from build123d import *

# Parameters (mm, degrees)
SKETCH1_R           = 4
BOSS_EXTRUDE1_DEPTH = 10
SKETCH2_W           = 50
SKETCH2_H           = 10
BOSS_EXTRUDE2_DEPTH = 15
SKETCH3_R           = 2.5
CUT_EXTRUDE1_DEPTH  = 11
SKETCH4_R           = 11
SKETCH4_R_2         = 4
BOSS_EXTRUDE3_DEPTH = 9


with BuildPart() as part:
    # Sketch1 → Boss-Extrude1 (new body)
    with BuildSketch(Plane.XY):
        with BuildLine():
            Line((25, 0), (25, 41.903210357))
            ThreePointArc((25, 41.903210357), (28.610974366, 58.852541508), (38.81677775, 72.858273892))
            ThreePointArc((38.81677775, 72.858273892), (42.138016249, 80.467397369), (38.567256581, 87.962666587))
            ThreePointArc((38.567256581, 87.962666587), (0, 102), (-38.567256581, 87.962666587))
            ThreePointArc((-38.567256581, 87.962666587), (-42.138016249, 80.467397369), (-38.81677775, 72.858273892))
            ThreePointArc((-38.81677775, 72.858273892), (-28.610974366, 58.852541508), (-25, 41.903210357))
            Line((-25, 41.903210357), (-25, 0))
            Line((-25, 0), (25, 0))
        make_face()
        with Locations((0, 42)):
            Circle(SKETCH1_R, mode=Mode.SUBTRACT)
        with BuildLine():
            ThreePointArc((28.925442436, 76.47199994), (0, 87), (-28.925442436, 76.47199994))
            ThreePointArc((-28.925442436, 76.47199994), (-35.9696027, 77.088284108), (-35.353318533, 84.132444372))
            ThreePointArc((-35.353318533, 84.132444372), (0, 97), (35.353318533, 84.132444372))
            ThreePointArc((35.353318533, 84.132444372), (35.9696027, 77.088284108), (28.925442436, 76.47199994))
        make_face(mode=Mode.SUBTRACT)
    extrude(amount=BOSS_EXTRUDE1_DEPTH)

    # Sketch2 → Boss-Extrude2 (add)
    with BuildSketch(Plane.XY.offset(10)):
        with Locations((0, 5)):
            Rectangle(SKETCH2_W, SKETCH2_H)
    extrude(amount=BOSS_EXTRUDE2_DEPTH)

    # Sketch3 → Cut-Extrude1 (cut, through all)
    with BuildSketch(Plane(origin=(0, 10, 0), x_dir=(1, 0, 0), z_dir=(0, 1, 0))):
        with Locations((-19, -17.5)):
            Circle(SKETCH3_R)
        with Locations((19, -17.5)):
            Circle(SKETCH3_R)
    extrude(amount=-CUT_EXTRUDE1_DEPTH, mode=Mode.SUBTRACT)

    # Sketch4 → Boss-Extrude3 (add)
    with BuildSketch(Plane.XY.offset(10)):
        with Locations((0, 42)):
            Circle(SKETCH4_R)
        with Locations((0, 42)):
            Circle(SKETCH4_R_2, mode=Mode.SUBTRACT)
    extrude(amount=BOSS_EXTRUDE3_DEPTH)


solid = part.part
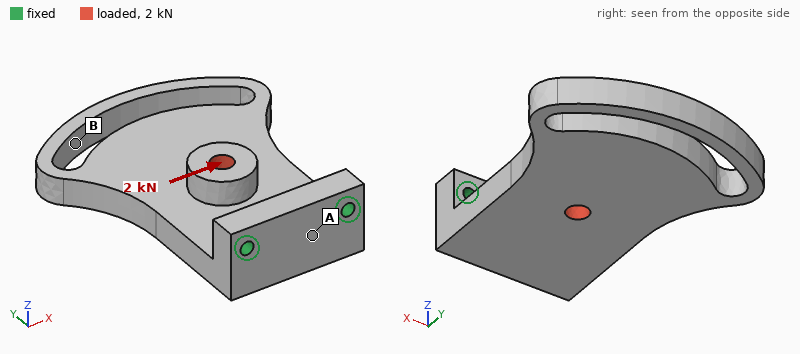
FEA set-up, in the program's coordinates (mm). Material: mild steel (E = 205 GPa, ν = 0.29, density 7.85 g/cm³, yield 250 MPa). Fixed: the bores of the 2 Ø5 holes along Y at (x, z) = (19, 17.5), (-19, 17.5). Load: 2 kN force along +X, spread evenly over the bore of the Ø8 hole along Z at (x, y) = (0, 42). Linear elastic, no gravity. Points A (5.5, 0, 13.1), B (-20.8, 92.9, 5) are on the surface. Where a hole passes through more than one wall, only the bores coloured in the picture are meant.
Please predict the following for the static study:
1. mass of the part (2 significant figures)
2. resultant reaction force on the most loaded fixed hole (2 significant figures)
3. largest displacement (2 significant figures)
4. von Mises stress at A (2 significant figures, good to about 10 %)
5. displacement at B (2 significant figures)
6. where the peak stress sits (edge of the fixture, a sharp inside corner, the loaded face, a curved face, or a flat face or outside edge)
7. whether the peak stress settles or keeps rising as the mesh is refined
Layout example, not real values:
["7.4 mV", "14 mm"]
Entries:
["480 g", "2.1 kN", "28 µm", "12 MPa", "25 µm", "edge of the fixture", "keeps rising"]
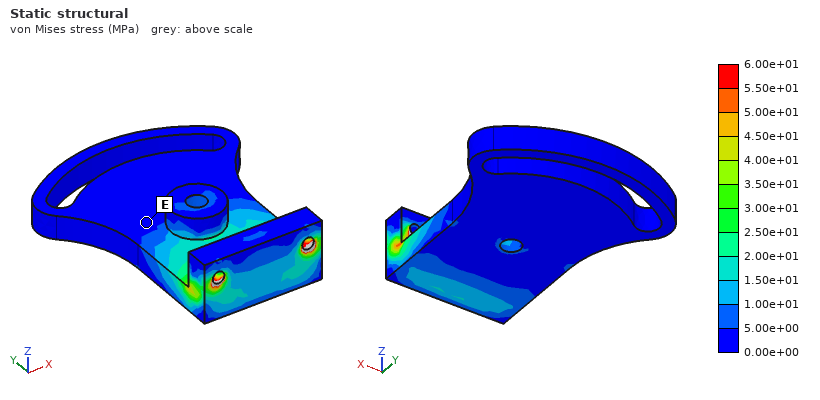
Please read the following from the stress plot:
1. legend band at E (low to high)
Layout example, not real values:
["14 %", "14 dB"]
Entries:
["0.00e+00 to 5.00e+00 MPa"]
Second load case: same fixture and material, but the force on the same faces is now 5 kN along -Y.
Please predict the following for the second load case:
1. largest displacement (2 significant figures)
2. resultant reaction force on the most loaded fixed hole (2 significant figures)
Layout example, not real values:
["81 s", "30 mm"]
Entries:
["34 µm", "2.5 kN"]
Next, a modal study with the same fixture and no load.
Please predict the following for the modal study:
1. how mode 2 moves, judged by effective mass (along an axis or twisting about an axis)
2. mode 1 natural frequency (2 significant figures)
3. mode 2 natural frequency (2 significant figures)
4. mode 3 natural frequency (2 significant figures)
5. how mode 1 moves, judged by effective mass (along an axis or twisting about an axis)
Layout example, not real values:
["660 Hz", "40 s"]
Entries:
["along X", "760 Hz", "2200 Hz", "2700 Hz", "along Z"]
